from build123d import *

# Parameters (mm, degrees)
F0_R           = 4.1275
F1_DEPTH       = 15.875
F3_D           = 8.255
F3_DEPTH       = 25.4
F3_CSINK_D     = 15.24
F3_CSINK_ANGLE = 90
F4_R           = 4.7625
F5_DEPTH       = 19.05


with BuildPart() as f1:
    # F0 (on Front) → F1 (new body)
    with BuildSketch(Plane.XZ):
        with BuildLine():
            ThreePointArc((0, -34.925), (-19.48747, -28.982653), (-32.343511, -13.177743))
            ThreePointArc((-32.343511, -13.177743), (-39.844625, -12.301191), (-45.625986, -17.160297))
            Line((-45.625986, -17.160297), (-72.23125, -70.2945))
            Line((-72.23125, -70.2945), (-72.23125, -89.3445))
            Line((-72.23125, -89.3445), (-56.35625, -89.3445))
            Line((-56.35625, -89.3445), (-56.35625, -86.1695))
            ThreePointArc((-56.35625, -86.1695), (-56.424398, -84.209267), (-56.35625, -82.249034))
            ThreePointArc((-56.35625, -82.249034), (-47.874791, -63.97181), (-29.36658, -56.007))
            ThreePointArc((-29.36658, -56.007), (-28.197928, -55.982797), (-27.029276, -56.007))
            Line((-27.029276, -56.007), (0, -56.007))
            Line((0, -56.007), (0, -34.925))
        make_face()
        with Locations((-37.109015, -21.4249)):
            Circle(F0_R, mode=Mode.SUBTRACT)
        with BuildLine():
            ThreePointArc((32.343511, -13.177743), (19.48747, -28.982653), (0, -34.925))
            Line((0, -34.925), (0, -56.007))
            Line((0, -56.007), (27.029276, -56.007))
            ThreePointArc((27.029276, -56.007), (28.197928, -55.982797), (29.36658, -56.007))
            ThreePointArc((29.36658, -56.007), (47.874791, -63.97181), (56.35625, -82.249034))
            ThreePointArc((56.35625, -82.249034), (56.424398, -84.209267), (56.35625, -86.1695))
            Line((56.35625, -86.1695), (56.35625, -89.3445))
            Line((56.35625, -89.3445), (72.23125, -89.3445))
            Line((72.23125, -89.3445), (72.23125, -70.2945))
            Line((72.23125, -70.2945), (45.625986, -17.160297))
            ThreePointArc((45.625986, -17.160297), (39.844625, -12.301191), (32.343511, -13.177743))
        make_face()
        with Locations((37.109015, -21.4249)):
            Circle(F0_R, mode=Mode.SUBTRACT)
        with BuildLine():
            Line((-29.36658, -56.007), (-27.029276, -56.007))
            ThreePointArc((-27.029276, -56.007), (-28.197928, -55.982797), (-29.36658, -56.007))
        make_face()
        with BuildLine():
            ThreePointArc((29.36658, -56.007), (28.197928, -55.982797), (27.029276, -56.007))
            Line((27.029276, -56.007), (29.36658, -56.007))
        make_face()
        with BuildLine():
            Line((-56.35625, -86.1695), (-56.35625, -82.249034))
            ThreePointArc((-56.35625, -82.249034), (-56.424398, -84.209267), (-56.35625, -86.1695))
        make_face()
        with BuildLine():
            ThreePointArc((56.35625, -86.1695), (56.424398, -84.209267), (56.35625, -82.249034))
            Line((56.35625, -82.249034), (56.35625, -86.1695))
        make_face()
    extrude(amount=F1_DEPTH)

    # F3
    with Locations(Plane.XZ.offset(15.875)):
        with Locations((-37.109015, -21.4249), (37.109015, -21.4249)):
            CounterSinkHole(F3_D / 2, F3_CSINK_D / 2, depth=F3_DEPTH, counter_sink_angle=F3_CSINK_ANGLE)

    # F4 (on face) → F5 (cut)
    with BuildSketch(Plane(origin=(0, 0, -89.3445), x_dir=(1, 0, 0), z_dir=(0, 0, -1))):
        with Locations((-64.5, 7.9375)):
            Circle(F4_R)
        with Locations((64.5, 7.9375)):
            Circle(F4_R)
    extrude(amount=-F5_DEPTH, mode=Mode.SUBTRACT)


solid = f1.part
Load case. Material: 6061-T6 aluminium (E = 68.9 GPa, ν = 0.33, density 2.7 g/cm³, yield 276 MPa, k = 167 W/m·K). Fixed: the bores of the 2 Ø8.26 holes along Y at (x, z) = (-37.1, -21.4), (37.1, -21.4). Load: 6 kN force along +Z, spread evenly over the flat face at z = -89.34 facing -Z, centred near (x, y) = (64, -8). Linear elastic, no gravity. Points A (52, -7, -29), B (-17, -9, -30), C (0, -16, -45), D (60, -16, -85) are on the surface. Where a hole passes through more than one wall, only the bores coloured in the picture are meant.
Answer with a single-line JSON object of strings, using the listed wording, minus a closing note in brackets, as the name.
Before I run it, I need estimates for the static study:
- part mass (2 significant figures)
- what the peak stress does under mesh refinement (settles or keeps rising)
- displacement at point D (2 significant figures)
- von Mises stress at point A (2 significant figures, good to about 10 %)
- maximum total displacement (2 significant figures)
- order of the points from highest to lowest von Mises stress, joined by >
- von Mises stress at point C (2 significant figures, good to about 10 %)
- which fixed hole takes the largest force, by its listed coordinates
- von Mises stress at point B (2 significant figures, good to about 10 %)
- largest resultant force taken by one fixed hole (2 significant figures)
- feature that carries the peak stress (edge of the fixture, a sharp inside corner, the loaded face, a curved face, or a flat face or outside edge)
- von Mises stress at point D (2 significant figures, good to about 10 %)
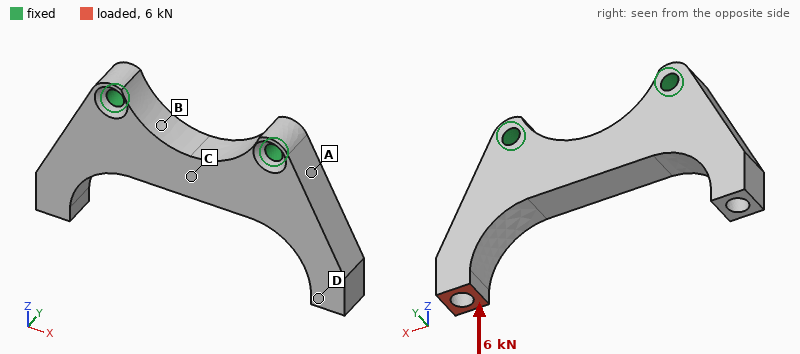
{"part mass": "200 g", "what the peak stress does under mesh refinement": "keeps rising", "displacement at point D": "0.14 mm", "von Mises stress at point A": "54 MPa", "maximum total displacement": "0.18 mm", "order of the points from highest to lowest von Mises stress, joined by >": "A > D > B > C", "von Mises stress at point C": "14 MPa", "which fixed hole takes the largest force, by its listed coordinates": "(37.1, -21.4)", "von Mises stress at point B": "23 MPa", "largest resultant force taken by one fixed hole": "8.1 kN", "feature that carries the peak stress": "edge of the fixture", "von Mises stress at point D": "32 MPa"}
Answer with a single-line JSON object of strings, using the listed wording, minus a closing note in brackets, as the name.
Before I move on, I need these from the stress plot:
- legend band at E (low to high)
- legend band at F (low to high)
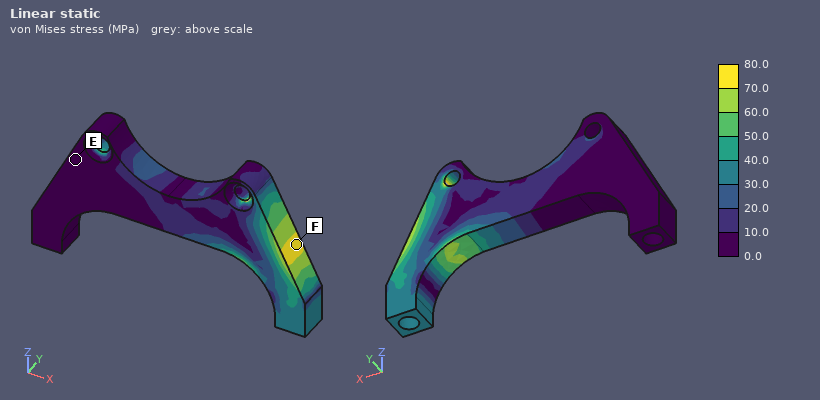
{"legend band at E": "0.0 to 10.0 MPa", "legend band at F": "70.0 to 80.0 MPa"}
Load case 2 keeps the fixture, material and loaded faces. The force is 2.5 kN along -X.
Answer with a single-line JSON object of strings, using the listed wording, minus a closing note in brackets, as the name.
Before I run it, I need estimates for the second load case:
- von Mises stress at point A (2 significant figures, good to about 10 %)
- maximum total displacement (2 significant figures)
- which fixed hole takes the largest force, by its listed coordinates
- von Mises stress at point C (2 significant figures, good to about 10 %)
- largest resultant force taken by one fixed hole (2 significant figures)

{"von Mises stress at point A": "33 MPa", "maximum total displacement": "0.22 mm", "which fixed hole takes the largest force, by its listed coordinates": "(-37.1, -21.4)", "von Mises stress at point C": "16 MPa", "largest resultant force taken by one fixed hole": "3.4 kN"}
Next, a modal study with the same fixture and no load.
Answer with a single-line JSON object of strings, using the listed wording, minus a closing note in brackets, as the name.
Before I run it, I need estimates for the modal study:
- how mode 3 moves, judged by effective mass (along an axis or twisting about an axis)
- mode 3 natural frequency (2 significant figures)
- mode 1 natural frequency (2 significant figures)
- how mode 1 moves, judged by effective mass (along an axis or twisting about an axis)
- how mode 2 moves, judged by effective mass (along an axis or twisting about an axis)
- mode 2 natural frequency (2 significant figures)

{"how mode 3 moves, judged by effective mass": "along X", "mode 3 natural frequency": "5400 Hz", "mode 1 natural frequency": "2800 Hz", "how mode 1 moves, judged by effective mass": "along Y", "how mode 2 moves, judged by effective mass": "twisting about Z", "mode 2 natural frequency": "3000 Hz"}
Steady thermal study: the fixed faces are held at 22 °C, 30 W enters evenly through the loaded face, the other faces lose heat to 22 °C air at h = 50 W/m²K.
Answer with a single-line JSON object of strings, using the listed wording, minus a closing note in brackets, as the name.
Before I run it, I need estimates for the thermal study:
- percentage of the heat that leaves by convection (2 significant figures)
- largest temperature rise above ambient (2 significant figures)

{"percentage of the heat that leaves by convection": "18 %", "largest temperature rise above ambient": "40 K"}
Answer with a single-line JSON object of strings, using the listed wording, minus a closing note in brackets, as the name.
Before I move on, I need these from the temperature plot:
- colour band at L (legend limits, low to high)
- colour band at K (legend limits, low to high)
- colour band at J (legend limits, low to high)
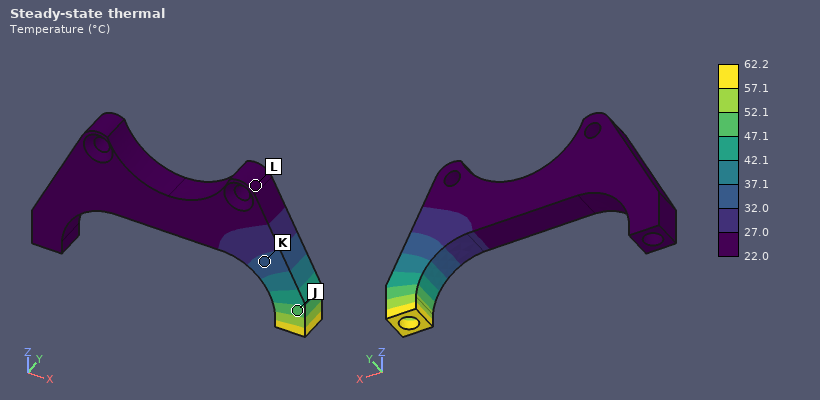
{"colour band at L": "22.0 to 27.0 °C", "colour band at K": "32.0 to 37.1 °C", "colour band at J": "47.1 to 52.1 °C"}
